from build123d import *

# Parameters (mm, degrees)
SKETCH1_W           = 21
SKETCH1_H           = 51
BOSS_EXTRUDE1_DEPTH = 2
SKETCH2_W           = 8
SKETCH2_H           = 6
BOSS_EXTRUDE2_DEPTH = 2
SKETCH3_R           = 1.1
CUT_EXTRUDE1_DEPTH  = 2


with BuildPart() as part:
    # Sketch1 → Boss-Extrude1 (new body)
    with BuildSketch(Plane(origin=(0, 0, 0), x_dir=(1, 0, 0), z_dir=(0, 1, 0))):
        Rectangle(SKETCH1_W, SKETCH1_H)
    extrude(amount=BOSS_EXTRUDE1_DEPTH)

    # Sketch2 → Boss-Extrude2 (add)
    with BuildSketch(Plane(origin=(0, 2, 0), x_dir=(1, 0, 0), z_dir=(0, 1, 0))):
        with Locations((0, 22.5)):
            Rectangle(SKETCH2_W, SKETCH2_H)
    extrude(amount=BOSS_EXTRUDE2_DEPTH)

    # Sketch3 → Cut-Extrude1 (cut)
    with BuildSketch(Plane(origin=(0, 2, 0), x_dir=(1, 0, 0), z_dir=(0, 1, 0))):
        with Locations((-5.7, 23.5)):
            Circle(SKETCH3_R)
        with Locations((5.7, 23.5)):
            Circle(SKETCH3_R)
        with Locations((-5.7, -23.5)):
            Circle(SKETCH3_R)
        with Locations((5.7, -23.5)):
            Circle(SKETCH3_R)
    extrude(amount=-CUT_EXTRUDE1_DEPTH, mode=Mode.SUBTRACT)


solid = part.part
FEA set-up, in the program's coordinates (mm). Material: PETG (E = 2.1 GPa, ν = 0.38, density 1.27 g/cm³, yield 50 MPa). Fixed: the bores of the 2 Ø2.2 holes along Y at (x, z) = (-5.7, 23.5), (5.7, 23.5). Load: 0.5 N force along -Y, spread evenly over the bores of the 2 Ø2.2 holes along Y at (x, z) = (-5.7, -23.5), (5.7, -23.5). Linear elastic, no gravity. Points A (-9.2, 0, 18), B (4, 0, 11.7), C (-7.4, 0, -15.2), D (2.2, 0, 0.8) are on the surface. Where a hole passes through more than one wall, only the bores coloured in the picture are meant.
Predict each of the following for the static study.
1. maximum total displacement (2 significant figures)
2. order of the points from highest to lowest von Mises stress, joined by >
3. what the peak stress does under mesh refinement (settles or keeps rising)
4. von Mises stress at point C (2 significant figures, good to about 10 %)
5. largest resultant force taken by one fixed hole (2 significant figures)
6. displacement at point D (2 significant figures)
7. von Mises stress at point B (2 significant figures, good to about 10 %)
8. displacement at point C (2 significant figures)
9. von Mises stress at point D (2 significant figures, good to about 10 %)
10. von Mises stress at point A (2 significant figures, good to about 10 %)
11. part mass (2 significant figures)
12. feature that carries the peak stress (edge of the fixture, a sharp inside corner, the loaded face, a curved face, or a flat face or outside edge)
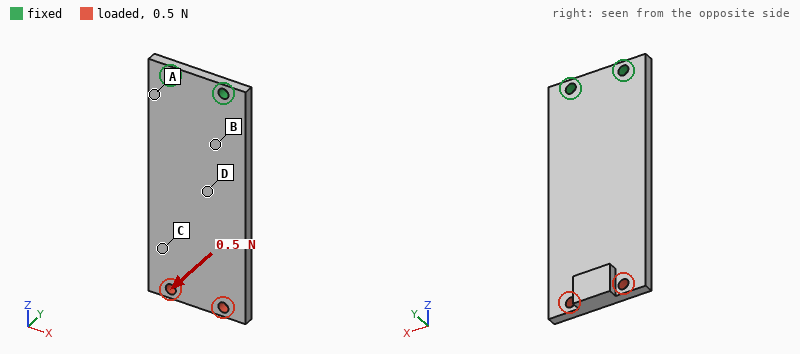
0.61 mm
A > B > D > C
keeps rising
0.31 MPa
0.25 N
0.17 mm
1.2 MPa
0.42 mm
0.85 MPa
1.5 MPa
2.8 g
edge of the fixture
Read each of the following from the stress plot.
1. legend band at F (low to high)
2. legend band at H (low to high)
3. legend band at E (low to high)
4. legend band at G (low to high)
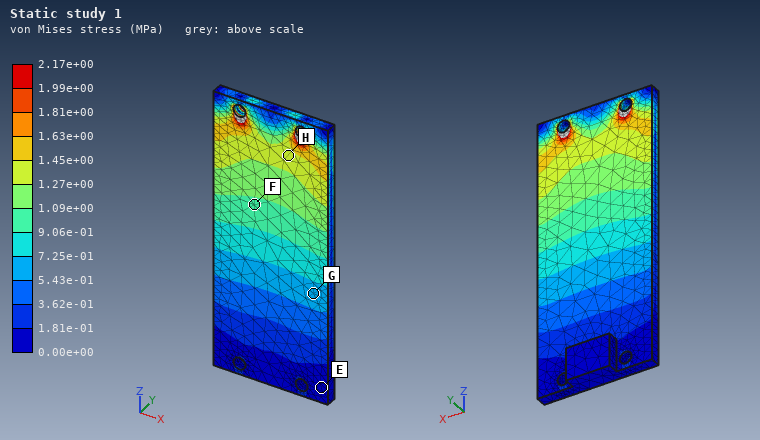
9.06e-01 to 1.09e+00 MPa
1.27e+00 to 1.45e+00 MPa
0.00e+00 to 1.81e-01 MPa
5.43e-01 to 7.25e-01 MPa
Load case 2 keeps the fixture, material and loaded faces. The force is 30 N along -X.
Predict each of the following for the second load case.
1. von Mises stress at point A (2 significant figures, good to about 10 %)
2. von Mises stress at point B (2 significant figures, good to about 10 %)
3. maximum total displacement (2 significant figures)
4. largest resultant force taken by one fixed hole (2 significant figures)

6.3 MPa
3.4 MPa
0.50 mm
110 N
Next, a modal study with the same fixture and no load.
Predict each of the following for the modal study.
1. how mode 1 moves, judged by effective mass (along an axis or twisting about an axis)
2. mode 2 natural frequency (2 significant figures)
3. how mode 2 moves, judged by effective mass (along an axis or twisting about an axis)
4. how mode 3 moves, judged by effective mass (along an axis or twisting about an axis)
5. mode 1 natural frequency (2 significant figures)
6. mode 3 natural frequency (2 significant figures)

along Y
810 Hz
twisting about Z
along Y
160 Hz
1100 Hz
